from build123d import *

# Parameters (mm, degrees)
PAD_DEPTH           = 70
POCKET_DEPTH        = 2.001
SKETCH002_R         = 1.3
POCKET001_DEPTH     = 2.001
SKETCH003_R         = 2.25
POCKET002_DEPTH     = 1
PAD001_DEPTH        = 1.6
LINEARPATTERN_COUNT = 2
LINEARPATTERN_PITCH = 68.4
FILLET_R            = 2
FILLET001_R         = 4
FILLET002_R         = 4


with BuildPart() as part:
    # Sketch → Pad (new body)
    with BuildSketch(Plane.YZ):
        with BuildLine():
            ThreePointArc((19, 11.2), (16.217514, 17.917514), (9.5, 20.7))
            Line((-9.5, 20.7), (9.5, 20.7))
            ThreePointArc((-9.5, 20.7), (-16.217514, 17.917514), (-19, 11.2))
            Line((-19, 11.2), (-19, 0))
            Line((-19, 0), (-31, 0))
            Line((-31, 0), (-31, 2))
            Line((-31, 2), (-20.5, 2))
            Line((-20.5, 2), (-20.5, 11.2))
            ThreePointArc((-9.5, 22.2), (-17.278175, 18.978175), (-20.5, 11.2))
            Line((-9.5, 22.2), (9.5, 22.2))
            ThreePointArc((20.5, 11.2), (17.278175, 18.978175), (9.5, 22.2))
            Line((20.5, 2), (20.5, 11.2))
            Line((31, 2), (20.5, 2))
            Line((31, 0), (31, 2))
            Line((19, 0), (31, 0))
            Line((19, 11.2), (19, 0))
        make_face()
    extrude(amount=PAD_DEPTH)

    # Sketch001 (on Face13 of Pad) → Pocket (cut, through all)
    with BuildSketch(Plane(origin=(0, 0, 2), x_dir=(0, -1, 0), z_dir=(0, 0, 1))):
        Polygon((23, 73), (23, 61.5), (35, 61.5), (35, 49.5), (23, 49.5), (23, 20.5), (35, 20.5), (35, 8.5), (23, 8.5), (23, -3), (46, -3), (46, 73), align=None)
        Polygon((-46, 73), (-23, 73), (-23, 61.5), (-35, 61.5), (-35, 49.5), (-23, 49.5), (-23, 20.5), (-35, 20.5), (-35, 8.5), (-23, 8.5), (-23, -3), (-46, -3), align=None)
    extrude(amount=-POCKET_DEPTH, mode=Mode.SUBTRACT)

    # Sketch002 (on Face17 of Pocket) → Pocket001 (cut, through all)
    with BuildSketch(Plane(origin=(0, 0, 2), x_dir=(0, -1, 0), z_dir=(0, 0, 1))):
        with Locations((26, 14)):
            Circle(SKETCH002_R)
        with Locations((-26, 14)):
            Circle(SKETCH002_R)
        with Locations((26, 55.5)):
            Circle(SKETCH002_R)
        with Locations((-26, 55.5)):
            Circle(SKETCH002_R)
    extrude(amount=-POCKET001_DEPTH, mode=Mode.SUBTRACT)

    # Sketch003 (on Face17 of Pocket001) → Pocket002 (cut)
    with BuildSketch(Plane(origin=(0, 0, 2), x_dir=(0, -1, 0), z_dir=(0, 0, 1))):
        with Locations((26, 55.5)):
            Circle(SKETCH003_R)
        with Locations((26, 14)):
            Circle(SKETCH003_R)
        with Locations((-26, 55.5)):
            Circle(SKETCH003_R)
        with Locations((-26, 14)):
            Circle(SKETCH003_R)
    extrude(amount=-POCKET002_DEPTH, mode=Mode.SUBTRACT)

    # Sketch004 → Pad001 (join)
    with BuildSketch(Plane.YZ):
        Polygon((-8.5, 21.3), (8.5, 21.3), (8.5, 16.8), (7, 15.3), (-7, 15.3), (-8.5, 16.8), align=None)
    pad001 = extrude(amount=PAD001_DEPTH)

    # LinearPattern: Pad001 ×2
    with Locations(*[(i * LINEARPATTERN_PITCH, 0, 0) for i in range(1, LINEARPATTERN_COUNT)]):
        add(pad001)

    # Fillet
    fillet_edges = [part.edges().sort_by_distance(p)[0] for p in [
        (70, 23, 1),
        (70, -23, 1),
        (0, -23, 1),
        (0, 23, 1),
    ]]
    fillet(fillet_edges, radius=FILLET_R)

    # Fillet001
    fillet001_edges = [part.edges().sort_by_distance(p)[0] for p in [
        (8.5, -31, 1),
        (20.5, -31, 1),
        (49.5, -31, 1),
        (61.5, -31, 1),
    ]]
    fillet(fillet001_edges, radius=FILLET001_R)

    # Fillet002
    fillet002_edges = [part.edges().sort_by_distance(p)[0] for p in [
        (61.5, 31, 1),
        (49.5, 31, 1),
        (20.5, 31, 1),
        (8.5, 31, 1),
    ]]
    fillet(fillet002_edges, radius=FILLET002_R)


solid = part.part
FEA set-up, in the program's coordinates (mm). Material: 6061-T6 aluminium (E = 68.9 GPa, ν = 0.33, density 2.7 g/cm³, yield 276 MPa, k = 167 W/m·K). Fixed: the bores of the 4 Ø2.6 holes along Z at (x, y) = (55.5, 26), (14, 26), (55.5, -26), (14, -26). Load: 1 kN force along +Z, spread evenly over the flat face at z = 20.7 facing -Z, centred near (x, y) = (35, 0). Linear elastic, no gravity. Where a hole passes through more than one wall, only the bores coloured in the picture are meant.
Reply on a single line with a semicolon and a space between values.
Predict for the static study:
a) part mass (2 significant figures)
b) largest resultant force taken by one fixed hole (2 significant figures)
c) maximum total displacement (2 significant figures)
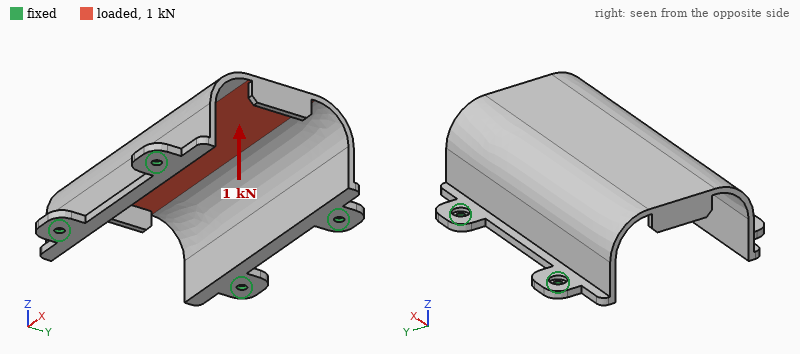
25 g; 300 N; 0.19 mm
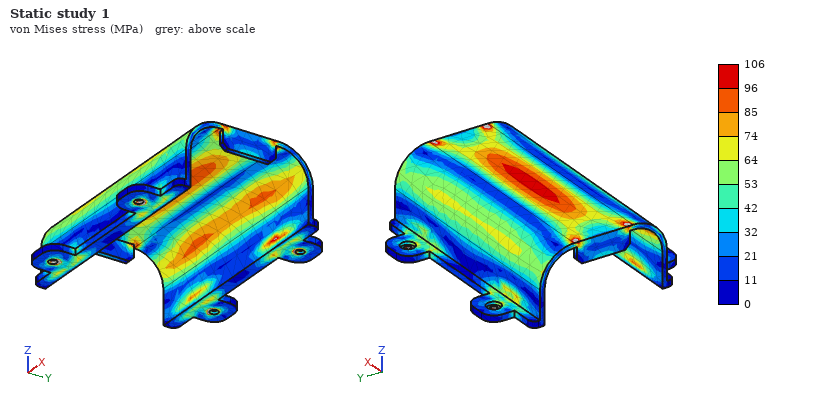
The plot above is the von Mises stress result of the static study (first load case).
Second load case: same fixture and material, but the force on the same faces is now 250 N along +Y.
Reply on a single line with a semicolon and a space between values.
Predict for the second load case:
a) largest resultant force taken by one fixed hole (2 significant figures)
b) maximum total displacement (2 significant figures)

75 N; 0.15 mm
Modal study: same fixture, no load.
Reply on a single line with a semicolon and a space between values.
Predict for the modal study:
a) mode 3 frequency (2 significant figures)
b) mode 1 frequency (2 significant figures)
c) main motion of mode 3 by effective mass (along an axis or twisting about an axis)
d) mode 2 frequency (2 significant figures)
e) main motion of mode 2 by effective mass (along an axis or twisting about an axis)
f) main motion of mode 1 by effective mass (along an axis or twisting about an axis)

4100 Hz; 1800 Hz; along X; 3400 Hz; twisting about Z; along Y
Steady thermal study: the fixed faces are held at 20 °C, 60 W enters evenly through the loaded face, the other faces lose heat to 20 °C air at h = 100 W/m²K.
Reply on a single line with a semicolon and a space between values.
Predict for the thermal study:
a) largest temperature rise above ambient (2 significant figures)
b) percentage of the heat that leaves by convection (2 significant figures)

53 K; 54 %
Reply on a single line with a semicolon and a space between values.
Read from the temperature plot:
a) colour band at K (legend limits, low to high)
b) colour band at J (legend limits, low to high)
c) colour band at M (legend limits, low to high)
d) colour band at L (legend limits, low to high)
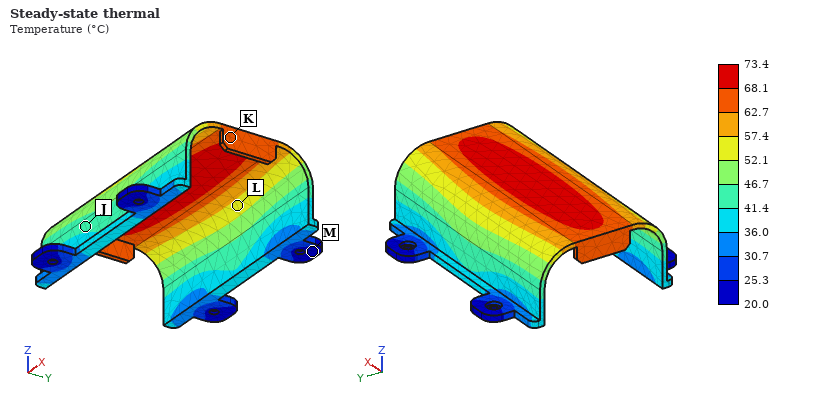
62.7 to 68.1 °C; 41.4 to 46.7 °C; 20.0 to 25.3 °C; 52.1 to 57.4 °C
